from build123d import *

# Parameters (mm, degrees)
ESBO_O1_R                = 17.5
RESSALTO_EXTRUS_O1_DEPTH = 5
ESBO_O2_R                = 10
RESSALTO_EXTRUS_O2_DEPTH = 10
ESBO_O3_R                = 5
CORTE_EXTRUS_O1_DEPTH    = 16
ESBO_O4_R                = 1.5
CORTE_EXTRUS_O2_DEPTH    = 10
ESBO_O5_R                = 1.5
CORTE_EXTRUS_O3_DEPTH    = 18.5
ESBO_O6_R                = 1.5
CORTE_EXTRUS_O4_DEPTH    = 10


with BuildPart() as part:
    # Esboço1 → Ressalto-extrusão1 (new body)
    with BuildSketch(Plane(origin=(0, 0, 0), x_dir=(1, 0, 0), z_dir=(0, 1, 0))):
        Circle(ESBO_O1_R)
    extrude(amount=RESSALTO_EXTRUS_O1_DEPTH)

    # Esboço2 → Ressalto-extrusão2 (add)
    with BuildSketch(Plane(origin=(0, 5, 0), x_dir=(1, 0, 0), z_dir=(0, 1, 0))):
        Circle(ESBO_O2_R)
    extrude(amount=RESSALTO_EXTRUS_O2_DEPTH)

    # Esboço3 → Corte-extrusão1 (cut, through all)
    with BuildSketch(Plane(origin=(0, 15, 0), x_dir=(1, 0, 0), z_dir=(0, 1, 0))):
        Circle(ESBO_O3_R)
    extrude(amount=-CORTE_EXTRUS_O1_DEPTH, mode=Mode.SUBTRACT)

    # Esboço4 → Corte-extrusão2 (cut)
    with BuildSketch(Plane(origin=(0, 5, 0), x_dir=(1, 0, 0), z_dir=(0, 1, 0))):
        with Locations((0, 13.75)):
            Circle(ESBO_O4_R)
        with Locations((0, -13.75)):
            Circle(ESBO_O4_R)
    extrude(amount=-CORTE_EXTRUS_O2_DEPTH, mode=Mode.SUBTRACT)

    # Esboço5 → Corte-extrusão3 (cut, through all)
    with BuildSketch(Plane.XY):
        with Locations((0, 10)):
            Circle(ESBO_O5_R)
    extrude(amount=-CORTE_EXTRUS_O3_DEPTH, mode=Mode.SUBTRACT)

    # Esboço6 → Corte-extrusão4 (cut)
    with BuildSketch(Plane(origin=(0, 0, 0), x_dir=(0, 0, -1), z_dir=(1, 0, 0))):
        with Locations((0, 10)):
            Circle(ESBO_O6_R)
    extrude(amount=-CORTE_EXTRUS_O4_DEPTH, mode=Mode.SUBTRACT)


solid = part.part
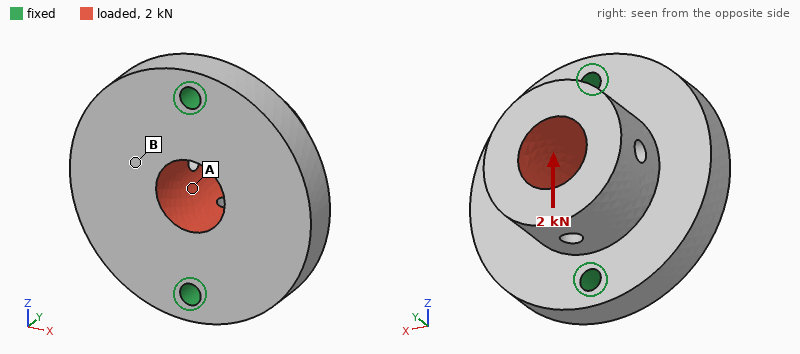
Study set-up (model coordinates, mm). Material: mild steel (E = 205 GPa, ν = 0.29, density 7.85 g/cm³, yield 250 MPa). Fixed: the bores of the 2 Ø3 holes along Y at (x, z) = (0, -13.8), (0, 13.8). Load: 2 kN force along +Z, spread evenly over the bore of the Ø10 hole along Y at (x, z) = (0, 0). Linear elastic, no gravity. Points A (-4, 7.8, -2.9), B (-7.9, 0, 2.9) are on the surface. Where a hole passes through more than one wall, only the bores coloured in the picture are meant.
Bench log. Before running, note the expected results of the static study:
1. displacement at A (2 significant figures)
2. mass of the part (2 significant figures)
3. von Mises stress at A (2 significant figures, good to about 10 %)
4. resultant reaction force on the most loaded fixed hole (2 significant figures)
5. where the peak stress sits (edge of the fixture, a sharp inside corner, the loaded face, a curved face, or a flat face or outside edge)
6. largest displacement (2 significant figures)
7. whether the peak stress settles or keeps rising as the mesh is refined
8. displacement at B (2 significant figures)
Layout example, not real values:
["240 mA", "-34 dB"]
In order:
["1.3 µm", "52 g", "14 MPa", "1.1 kN", "edge of the fixture", "2.4 µm", "keeps rising", "0.62 µm"]
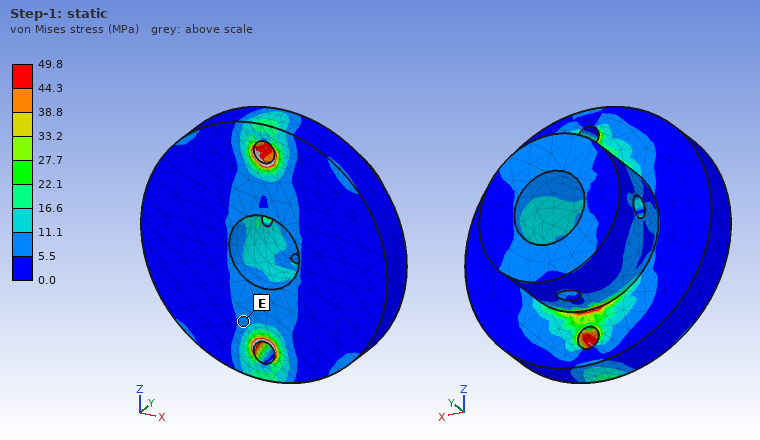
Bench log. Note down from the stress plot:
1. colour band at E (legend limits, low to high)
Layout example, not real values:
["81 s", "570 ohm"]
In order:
["5.5 to 11.1 MPa"]
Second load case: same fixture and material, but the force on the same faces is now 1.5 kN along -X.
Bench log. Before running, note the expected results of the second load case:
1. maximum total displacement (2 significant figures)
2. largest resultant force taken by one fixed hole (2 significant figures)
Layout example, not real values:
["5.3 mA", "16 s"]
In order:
["9.0 µm", "750 N"]
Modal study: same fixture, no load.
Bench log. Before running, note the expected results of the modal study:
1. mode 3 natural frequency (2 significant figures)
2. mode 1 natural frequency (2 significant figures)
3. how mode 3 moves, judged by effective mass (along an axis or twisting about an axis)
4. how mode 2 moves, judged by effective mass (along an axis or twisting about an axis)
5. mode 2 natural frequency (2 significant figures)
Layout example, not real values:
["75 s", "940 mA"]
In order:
["29 kHz", "9300 Hz", "along Z", "along Y", "18 kHz"]
